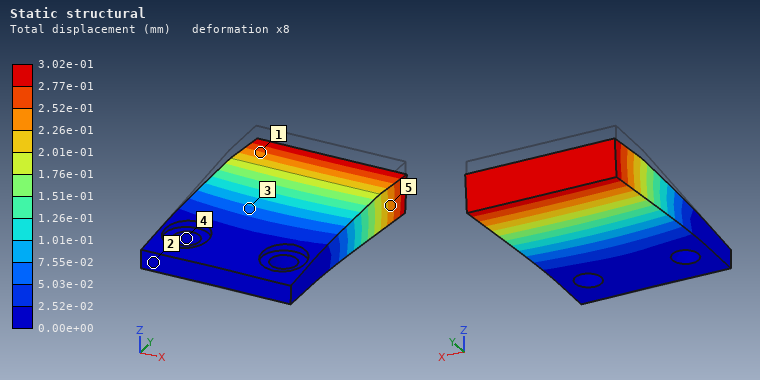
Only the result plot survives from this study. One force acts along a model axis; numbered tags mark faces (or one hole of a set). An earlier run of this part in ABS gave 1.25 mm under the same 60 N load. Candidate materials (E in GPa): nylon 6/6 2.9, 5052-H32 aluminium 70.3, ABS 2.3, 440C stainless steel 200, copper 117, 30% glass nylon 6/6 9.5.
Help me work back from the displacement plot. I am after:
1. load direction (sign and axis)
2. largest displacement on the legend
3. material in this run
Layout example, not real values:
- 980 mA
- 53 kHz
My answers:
- -Z
- 3.02e-01 mm
- 30% glass nylon 6/6
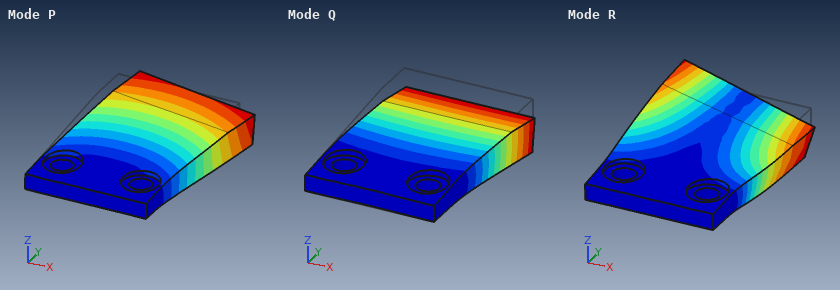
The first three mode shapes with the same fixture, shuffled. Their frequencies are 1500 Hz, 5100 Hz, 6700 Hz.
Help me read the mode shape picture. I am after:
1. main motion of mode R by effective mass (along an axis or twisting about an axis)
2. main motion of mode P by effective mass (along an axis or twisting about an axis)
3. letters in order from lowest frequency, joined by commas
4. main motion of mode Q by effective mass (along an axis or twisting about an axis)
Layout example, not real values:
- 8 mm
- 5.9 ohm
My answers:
- twisting about Y
- along X
- Q, R, P
- along Z
